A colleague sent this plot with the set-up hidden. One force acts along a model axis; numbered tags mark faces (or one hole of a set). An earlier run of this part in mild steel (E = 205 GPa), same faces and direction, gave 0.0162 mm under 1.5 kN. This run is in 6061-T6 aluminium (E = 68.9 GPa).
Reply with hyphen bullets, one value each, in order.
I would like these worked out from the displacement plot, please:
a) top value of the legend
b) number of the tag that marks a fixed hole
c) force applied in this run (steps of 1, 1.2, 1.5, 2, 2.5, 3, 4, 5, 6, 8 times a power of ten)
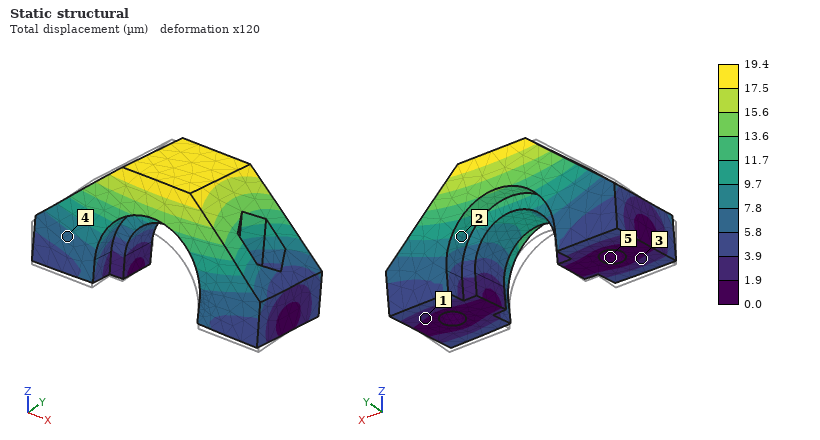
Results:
- 19.4 µm
- 5
- 600 N
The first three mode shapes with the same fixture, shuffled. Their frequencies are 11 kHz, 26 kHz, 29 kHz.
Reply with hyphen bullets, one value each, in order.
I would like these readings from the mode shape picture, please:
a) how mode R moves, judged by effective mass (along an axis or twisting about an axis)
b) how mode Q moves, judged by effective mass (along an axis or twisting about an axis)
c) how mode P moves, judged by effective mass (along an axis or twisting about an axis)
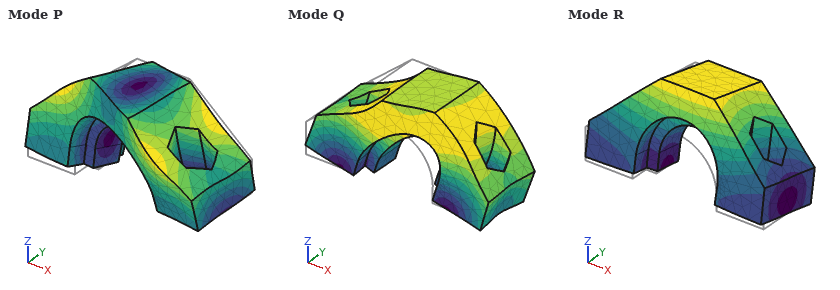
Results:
- along Y
- along X
- twisting about Z
